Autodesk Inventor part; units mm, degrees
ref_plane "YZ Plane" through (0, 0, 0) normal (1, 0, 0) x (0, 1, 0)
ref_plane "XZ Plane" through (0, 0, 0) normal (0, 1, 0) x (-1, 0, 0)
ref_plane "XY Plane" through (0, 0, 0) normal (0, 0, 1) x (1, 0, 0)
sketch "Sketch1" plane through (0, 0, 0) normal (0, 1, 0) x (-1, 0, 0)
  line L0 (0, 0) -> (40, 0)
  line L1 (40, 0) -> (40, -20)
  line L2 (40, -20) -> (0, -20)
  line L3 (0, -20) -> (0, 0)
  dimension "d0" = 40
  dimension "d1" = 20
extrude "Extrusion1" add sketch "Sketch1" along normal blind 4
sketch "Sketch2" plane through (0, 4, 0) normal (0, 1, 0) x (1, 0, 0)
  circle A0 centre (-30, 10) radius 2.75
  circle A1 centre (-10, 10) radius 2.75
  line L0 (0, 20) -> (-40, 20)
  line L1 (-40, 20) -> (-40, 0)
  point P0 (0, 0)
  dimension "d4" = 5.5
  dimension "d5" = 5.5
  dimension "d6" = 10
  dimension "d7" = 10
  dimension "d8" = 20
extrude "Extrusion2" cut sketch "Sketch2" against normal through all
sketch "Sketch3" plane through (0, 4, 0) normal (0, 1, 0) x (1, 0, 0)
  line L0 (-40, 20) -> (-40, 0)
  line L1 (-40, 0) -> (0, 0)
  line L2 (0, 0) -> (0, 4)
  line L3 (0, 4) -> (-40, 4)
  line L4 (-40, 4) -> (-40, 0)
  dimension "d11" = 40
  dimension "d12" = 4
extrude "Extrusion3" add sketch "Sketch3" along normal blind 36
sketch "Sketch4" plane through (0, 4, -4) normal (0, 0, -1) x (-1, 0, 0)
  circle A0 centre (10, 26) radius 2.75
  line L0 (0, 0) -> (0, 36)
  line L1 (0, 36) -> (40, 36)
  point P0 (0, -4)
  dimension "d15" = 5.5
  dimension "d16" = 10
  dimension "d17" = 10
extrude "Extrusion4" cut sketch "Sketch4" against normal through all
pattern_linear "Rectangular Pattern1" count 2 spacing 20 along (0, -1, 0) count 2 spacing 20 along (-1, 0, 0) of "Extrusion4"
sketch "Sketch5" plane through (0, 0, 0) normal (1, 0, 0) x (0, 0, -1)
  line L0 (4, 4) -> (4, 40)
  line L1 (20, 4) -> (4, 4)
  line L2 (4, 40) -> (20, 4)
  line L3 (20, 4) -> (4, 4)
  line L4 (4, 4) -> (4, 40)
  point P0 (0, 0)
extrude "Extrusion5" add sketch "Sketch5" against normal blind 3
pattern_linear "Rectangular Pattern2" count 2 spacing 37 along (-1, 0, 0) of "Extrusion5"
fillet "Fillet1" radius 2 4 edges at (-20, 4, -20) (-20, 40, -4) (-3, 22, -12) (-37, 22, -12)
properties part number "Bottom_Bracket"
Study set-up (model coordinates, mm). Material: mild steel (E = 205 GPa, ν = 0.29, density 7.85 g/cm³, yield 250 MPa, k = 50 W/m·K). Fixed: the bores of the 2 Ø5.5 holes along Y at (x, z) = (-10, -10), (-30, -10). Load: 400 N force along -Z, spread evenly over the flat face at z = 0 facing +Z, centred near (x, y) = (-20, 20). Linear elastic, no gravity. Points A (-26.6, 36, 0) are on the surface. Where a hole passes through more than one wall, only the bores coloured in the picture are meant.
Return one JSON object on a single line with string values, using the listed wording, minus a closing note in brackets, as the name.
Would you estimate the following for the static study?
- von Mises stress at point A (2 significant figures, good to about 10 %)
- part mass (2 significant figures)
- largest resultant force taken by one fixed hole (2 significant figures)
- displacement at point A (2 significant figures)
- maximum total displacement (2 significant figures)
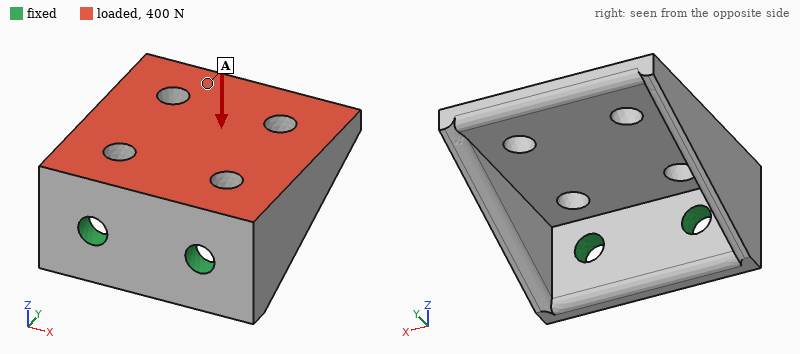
{"von Mises stress at point A": "12 MPa", "part mass": "78 g", "largest resultant force taken by one fixed hole": "200 N", "displacement at point A": "22 µm", "maximum total displacement": "26 µm"}
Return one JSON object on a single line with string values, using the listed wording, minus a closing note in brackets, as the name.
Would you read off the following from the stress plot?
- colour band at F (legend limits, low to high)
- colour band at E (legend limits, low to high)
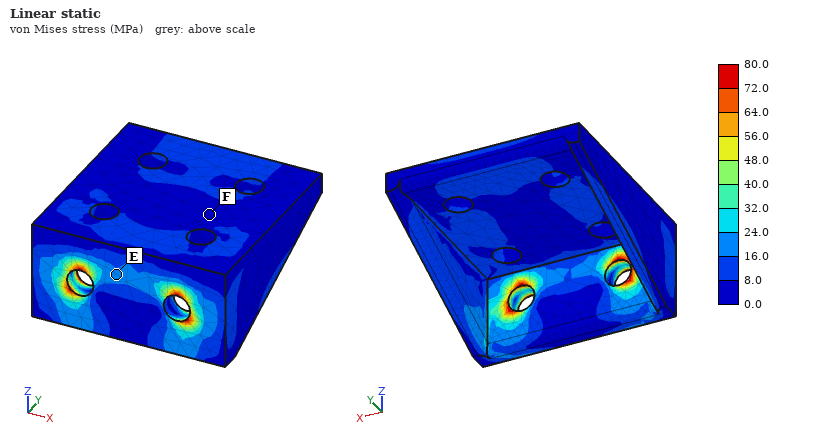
{"colour band at F": "0.0 to 8.0 MPa", "colour band at E": "16.0 to 24.0 MPa"}
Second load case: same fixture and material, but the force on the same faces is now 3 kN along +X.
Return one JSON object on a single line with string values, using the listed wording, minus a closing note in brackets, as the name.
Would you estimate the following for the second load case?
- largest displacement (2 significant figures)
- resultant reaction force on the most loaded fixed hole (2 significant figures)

{"largest displacement": "46 µm", "resultant reaction force on the most loaded fixed hole": "2.7 kN"}
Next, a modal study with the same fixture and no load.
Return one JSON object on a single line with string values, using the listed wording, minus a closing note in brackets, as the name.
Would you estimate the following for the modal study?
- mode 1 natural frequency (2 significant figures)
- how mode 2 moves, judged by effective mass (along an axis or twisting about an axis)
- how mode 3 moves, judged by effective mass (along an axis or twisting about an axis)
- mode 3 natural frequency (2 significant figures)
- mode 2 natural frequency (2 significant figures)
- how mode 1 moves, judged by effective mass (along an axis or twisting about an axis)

{"mode 1 natural frequency": "3400 Hz", "how mode 2 moves, judged by effective mass": "along X", "how mode 3 moves, judged by effective mass": "along X", "mode 3 natural frequency": "9200 Hz", "mode 2 natural frequency": "5000 Hz", "how mode 1 moves, judged by effective mass": "along Z"}
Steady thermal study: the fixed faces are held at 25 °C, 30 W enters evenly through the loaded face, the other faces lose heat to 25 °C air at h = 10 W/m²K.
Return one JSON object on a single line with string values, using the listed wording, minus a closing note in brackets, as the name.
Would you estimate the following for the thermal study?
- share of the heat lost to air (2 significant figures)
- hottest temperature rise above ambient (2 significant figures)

{"share of the heat lost to air": "5.5 %", "hottest temperature rise above ambient": "72 K"}
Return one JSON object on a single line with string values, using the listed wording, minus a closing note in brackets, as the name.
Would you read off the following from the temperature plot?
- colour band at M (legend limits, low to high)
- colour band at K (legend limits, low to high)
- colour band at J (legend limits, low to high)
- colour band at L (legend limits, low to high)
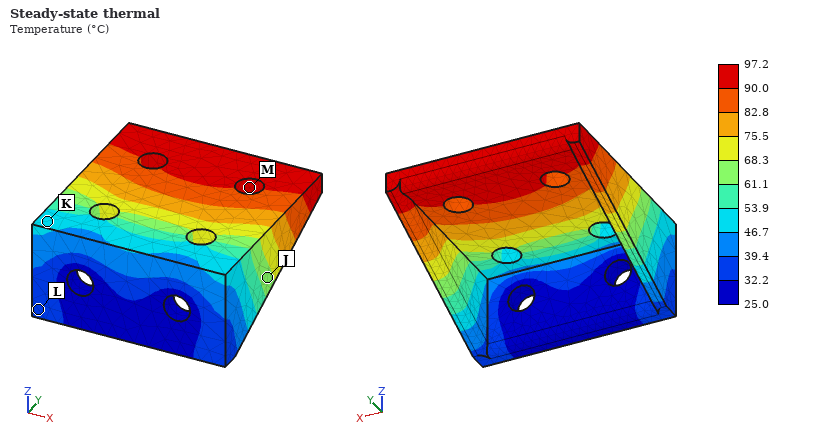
{"colour band at M": "90.0 to 97.2 °C", "colour band at K": "46.7 to 53.9 °C", "colour band at J": "61.1 to 68.3 °C", "colour band at L": "32.2 to 39.4 °C"}
